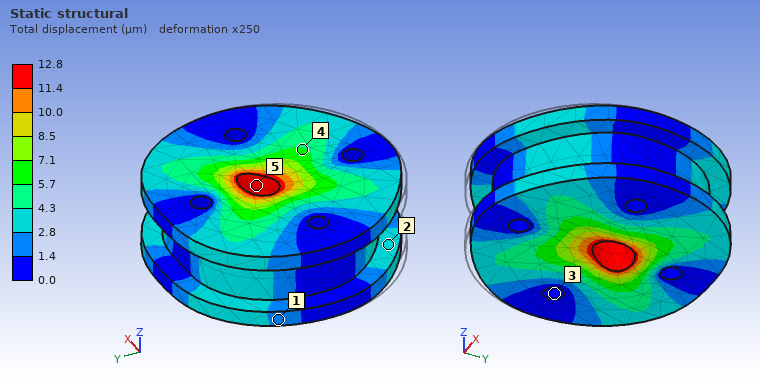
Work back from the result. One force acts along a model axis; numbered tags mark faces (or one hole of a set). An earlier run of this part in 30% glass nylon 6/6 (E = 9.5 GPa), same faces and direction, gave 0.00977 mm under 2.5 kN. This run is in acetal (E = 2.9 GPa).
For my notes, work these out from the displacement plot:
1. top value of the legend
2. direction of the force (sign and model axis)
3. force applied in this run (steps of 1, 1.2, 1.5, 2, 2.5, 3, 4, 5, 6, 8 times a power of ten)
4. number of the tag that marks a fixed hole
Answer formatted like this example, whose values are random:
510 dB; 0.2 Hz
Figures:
12.8 µm; +Y; 1 kN; 3
